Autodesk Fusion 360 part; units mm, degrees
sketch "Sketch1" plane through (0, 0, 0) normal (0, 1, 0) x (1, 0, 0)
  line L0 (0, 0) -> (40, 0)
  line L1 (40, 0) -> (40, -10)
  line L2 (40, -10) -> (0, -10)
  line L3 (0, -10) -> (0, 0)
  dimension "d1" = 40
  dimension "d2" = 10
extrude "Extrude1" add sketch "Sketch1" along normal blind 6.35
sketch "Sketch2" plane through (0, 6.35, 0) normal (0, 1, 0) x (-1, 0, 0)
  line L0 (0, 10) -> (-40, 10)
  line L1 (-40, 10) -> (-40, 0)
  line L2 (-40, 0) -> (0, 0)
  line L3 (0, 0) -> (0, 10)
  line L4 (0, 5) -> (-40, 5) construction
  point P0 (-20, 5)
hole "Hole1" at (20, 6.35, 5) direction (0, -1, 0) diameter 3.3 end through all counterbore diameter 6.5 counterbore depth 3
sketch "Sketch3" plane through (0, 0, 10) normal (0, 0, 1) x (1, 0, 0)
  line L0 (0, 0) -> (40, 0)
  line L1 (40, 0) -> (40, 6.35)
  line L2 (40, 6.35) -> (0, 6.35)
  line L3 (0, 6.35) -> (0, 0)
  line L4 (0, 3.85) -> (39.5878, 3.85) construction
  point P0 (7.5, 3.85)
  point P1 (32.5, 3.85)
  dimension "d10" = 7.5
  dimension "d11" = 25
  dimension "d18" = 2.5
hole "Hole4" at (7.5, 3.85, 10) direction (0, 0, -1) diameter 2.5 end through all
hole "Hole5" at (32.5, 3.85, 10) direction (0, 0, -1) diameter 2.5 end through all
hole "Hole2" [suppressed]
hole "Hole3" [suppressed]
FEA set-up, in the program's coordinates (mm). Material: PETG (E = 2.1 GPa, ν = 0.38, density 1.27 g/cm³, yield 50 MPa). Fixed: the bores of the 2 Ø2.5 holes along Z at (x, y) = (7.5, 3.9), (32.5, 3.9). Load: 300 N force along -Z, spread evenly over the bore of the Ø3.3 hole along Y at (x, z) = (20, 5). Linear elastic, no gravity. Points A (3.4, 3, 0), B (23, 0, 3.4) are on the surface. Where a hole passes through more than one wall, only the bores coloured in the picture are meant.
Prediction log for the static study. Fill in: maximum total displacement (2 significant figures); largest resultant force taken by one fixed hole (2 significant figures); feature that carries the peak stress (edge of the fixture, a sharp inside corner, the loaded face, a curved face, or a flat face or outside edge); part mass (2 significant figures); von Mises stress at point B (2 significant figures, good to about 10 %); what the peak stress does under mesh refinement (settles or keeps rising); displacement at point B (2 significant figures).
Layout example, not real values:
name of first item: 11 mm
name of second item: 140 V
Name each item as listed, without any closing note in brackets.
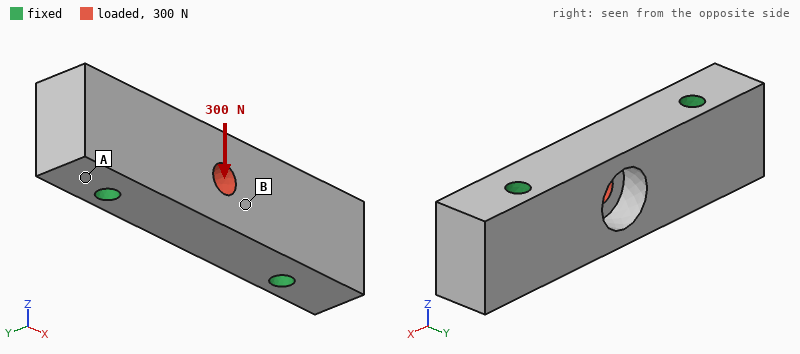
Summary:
maximum total displacement: 89 µm
largest resultant force taken by one fixed hole: 150 N
feature that carries the peak stress: edge of the fixture
part mass: 2.9 g
von Mises stress at point B: 8.8 MPa
what the peak stress does under mesh refinement: keeps rising
displacement at point B: 67 µm
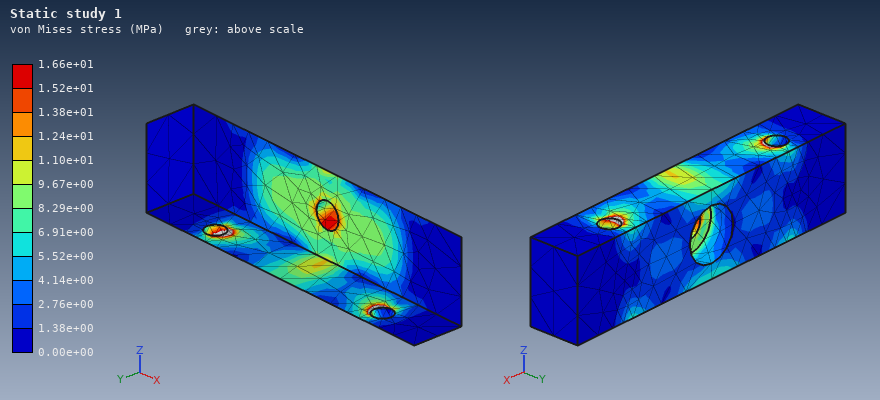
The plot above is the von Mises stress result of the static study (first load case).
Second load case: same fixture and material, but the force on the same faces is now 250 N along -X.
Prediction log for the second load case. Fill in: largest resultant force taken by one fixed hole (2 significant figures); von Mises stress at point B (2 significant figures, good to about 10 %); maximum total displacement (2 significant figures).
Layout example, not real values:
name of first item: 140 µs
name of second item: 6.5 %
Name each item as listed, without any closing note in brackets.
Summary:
largest resultant force taken by one fixed hole: 130 N
von Mises stress at point B: 5.6 MPa
maximum total displacement: 21 µm
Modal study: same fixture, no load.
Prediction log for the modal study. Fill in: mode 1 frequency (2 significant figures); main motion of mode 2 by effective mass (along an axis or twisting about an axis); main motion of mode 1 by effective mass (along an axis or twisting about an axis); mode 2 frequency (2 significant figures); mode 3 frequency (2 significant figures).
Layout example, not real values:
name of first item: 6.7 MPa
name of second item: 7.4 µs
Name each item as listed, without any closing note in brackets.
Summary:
mode 1 frequency: 9000 Hz
main motion of mode 2 by effective mass: along Z
main motion of mode 1 by effective mass: along Y
mode 2 frequency: 13 kHz
mode 3 frequency: 14 kHz
